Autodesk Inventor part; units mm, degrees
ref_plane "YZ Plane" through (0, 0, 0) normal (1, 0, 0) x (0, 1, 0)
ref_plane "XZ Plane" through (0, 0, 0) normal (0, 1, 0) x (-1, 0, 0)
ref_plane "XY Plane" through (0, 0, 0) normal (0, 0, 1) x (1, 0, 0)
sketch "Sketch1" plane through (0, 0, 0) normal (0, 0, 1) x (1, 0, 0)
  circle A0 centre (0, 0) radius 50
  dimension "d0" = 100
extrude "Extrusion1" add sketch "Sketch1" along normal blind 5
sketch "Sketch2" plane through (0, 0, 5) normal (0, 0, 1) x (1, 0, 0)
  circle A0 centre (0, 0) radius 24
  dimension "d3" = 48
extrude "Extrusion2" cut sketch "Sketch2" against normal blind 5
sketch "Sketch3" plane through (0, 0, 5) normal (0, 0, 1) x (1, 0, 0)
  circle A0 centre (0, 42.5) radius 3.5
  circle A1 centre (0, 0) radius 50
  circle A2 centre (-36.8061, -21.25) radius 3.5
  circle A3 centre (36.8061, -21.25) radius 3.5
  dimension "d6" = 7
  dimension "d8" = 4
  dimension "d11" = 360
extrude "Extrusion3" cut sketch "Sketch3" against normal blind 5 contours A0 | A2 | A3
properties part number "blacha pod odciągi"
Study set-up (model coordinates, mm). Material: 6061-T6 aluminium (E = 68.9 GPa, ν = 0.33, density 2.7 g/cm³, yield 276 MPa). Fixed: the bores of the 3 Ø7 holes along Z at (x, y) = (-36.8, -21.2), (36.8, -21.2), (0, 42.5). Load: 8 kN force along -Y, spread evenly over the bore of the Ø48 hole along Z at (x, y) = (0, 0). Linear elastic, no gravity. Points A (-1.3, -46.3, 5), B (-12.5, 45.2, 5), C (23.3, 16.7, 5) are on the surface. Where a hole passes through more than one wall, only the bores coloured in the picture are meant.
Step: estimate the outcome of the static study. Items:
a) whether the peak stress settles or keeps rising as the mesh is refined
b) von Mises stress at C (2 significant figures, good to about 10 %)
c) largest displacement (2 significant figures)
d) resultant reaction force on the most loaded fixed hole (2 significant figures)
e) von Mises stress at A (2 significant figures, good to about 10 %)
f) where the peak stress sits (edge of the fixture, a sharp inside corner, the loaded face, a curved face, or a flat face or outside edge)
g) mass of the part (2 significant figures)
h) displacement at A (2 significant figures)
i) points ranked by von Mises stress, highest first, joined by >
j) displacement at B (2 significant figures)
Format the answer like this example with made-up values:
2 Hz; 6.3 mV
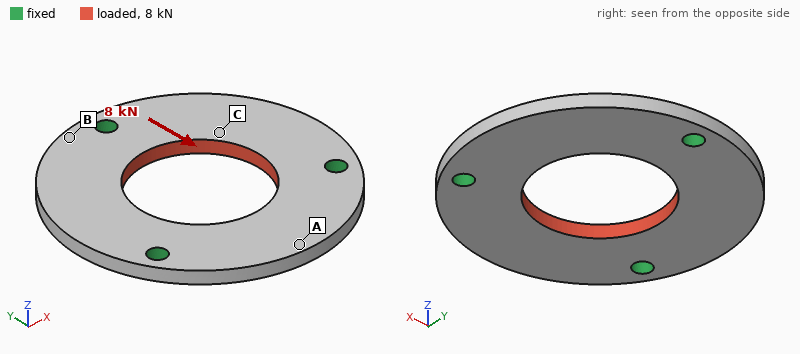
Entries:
keeps rising; 10.0 MPa; 18 µm; 3.0 kN; 17 MPa; edge of the fixture; 80 g; 15 µm; A > C > B; 4.0 µm
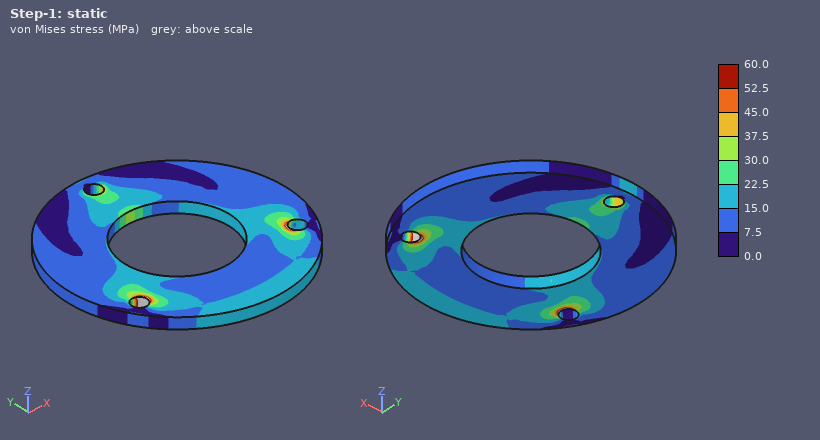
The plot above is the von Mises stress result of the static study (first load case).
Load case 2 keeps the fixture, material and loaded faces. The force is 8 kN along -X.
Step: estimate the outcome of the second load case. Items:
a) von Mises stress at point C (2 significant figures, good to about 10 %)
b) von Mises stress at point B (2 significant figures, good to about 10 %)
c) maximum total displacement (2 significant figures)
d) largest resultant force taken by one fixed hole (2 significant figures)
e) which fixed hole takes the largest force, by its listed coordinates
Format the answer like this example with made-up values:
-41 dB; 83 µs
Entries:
9.9 MPa; 14 MPa; 16 µm; 3.3 kN; (0, 42.5)
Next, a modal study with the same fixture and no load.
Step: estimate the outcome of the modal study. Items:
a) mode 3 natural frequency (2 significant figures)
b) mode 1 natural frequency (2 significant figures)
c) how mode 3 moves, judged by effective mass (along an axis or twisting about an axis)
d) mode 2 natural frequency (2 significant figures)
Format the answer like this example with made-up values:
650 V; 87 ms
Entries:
3600 Hz; 3400 Hz; along Z; 3400 Hz
